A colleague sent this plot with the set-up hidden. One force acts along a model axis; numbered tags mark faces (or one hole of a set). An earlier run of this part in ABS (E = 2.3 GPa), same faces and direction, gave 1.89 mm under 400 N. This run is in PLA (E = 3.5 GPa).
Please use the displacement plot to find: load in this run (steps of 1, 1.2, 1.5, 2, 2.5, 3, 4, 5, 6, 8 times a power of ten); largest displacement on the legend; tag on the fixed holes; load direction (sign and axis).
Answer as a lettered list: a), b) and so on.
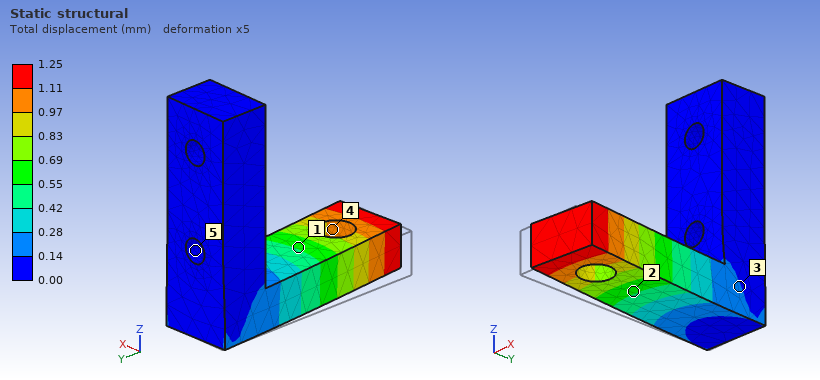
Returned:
a) 400 N
b) 1.25 mm
c) 5
d) +X
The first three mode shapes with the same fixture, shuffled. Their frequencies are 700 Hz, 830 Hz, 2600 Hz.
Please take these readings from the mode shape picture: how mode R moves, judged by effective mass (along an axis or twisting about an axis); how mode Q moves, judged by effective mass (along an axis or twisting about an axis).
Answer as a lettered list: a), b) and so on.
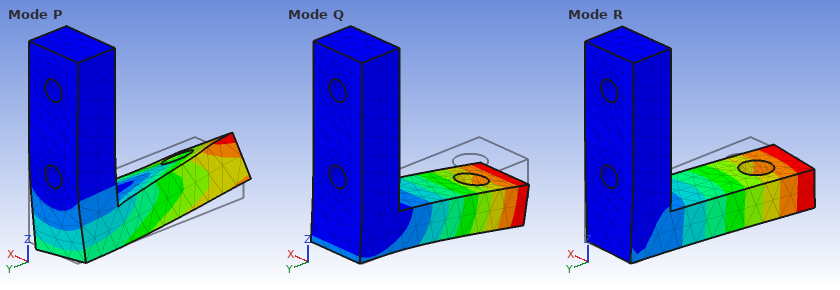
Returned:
a) along X
b) along Z
